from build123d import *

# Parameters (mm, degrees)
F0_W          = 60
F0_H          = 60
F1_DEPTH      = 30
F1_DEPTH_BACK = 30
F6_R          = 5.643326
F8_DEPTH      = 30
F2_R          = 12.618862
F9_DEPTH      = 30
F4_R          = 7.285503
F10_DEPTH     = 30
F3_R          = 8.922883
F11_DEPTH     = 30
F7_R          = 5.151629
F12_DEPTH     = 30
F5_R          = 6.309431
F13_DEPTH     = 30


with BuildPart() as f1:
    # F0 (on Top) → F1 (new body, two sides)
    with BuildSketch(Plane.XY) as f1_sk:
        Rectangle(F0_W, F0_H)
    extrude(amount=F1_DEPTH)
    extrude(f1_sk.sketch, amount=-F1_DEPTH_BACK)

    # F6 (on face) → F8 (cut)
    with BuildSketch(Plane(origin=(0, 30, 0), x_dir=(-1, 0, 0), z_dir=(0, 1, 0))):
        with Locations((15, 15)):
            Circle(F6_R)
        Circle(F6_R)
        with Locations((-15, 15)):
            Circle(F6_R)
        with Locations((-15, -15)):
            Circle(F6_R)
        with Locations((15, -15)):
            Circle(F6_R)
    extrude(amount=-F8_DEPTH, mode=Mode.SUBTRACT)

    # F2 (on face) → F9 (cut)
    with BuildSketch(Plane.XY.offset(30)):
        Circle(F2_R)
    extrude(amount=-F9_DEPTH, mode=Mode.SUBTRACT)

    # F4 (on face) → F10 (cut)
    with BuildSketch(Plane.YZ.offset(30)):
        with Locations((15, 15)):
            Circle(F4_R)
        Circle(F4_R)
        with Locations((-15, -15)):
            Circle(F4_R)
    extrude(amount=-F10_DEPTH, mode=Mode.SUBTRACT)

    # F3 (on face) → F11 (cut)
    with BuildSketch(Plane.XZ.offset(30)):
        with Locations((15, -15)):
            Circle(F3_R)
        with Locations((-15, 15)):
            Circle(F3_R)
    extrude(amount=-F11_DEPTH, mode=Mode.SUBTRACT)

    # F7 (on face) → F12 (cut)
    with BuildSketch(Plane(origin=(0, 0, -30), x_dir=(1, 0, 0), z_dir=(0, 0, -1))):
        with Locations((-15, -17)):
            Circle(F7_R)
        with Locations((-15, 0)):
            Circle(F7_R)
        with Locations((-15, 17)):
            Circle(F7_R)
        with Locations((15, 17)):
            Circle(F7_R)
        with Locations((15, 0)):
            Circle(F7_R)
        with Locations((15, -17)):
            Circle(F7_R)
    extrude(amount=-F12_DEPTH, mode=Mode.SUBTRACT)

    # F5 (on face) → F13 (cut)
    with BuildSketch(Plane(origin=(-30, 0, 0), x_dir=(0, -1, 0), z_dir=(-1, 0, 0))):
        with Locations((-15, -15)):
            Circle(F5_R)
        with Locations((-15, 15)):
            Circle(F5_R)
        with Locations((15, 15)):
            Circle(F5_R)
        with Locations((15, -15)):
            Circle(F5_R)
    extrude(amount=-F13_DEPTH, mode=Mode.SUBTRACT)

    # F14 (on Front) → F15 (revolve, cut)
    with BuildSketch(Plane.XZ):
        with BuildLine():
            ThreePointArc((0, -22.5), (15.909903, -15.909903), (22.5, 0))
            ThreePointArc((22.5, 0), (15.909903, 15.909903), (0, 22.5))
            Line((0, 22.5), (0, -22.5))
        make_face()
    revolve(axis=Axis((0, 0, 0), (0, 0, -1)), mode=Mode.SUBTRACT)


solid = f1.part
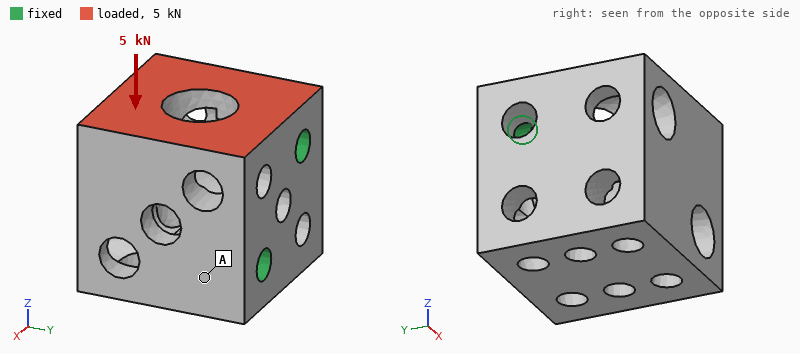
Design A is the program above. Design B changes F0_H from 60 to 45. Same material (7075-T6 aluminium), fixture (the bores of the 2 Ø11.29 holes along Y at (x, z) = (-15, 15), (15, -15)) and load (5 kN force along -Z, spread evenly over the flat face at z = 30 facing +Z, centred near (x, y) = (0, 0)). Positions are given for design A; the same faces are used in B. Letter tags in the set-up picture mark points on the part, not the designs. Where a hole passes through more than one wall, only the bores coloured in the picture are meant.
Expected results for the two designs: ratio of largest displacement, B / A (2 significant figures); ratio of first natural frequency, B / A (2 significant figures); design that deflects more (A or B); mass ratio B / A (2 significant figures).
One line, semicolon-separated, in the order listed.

1.9; 0.92; B; 0.62
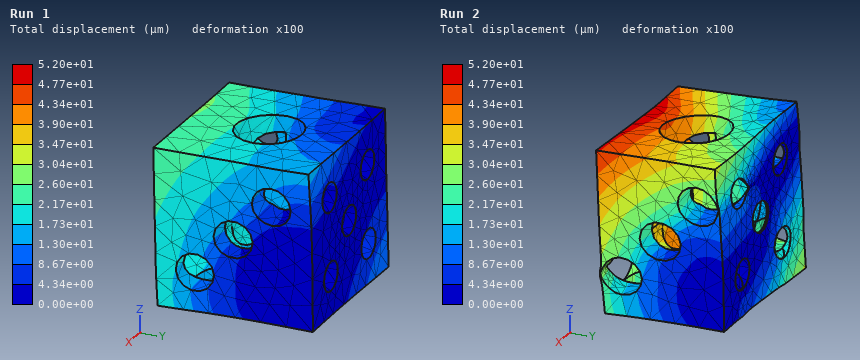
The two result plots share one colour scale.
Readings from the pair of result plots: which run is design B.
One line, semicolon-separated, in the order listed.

Run 2
